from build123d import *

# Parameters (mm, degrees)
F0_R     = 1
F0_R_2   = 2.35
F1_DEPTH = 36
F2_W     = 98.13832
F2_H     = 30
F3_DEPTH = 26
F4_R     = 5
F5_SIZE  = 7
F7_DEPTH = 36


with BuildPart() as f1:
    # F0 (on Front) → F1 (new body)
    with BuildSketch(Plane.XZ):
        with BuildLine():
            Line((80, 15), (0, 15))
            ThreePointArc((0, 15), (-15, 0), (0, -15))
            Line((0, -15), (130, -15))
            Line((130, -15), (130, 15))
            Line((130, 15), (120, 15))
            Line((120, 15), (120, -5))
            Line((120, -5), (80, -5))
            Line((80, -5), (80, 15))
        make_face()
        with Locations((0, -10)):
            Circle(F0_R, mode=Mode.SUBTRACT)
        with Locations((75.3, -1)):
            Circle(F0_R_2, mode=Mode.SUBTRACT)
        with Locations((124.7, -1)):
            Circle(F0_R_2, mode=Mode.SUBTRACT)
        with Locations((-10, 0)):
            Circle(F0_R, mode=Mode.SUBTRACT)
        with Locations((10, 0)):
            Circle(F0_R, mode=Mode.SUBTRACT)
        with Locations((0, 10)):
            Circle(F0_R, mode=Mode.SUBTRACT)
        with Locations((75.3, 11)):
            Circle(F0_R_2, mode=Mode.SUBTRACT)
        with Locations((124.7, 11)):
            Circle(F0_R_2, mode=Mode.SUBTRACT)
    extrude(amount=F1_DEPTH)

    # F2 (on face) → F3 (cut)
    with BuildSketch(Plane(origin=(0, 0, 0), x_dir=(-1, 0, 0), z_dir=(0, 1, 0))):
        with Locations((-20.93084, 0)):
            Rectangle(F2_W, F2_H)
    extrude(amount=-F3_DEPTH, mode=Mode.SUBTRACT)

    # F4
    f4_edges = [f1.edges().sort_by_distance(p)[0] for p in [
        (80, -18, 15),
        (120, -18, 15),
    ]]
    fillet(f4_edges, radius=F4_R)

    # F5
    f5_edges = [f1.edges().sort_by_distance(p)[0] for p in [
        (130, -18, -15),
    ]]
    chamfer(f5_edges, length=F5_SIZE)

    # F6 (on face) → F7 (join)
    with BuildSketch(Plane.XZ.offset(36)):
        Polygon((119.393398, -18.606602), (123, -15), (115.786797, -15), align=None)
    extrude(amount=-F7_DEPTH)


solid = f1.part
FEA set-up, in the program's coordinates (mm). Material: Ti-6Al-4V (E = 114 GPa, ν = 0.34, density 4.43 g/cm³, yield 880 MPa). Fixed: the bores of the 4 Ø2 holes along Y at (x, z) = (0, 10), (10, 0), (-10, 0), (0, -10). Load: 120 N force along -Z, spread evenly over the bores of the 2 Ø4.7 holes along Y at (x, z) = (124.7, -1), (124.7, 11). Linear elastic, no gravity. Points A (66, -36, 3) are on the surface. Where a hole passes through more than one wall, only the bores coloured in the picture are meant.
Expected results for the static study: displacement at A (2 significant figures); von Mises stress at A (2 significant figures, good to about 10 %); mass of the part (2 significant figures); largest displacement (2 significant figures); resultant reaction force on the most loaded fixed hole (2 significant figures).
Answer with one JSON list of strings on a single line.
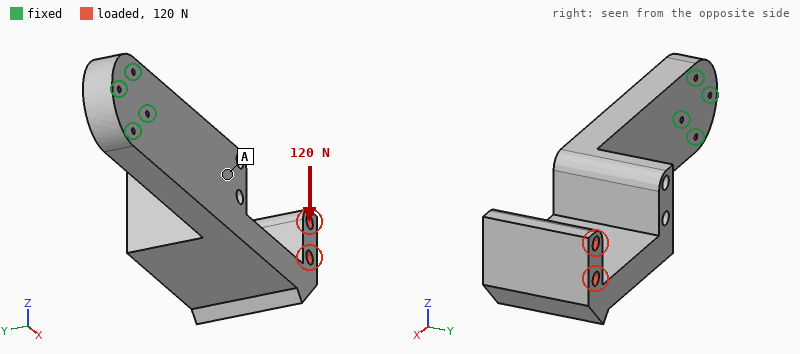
["10 µm", "1.2 MPa", "250 g", "65 µm", "500 N"]
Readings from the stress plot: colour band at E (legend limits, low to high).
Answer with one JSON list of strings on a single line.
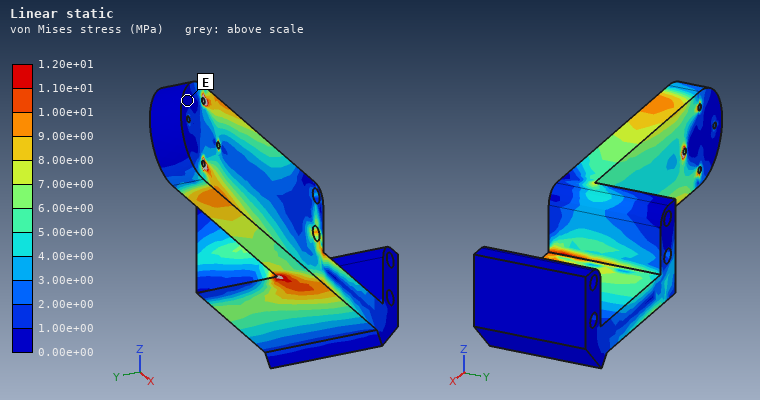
["0.00e+00 to 1.00e+00 MPa"]
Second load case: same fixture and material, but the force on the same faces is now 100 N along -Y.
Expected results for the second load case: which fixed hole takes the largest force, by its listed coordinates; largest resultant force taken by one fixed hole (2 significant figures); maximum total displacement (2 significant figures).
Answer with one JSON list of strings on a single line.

["(10, 0)", "560 N", "0.21 mm"]
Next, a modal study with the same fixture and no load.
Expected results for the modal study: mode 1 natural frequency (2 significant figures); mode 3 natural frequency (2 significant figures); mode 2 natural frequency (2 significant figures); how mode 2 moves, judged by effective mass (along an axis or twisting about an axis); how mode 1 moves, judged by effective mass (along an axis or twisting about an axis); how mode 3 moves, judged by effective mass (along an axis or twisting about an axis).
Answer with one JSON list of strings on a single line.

["390 Hz", "2000 Hz", "870 Hz", "along Z", "along Y", "twisting about X"]
